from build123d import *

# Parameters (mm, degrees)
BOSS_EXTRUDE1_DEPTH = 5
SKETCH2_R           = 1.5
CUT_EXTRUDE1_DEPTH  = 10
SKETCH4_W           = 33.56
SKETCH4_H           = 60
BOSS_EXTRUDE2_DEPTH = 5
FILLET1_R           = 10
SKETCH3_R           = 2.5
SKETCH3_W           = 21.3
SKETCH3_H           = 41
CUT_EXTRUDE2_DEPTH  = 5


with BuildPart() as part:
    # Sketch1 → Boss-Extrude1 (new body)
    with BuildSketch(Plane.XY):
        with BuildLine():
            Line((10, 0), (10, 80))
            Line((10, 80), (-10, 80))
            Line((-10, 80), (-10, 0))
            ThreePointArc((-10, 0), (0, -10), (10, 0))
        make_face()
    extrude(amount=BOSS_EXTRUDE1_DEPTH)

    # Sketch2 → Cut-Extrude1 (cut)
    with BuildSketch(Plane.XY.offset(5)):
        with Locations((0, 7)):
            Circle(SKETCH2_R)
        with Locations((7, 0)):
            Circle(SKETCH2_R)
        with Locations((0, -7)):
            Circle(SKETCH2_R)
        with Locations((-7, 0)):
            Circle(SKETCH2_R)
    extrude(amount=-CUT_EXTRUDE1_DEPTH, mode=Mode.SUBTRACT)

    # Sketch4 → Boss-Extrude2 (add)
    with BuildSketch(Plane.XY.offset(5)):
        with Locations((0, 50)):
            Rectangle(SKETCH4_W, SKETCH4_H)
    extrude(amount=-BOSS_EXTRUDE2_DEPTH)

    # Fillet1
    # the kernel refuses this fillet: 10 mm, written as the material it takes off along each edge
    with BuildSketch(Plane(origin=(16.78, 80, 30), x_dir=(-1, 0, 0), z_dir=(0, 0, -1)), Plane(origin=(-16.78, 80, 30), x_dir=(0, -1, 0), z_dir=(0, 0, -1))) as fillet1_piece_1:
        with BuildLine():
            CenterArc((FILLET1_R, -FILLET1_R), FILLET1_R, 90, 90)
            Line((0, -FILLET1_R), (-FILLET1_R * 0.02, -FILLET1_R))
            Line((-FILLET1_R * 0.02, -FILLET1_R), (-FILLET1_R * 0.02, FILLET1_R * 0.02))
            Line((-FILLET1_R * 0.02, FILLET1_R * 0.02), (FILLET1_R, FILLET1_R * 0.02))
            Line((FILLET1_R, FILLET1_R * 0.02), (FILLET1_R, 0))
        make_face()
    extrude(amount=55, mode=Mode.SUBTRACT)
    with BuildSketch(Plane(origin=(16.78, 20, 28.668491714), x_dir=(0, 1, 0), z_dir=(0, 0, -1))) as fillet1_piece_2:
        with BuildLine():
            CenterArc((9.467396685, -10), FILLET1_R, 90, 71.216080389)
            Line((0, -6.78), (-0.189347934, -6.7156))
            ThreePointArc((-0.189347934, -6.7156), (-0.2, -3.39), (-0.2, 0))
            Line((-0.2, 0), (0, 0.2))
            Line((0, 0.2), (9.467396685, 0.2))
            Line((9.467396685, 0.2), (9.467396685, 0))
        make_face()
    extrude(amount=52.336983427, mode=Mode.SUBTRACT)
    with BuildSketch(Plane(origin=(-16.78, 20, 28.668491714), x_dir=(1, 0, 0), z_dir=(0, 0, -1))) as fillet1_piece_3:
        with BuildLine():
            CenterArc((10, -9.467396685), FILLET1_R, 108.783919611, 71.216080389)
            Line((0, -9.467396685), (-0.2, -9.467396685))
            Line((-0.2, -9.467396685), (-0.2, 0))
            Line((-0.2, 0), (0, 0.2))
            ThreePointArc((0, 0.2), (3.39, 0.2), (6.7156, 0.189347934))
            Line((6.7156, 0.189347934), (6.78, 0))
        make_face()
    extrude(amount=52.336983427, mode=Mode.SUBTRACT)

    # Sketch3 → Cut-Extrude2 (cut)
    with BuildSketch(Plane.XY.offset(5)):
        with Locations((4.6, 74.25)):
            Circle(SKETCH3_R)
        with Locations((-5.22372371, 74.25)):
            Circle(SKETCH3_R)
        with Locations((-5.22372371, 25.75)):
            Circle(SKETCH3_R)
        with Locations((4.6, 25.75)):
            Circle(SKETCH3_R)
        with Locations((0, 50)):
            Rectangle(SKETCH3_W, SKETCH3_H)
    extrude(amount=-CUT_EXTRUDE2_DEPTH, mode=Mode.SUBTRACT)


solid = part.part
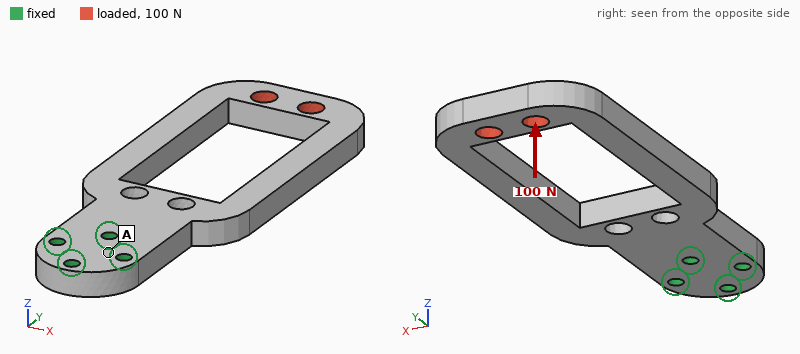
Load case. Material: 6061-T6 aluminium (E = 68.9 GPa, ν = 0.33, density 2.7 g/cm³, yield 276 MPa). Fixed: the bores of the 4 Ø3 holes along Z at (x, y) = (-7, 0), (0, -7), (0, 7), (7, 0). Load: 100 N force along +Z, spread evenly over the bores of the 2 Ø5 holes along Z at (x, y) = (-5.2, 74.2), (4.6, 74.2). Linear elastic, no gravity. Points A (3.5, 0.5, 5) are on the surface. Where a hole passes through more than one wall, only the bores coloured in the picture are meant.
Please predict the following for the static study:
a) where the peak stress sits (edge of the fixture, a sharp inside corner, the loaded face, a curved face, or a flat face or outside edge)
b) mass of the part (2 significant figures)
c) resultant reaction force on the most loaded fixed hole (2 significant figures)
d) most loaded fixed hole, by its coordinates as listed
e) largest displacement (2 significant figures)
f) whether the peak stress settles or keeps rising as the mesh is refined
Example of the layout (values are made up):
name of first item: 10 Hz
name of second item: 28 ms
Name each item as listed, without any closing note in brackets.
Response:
where the peak stress sits: edge of the fixture
mass of the part: 20 g
resultant reaction force on the most loaded fixed hole: 500 N
most loaded fixed hole, by its coordinates as listed: (0, 7)
largest displacement: 1.1 mm
whether the peak stress settles or keeps rising as the mesh is refined: keeps rising
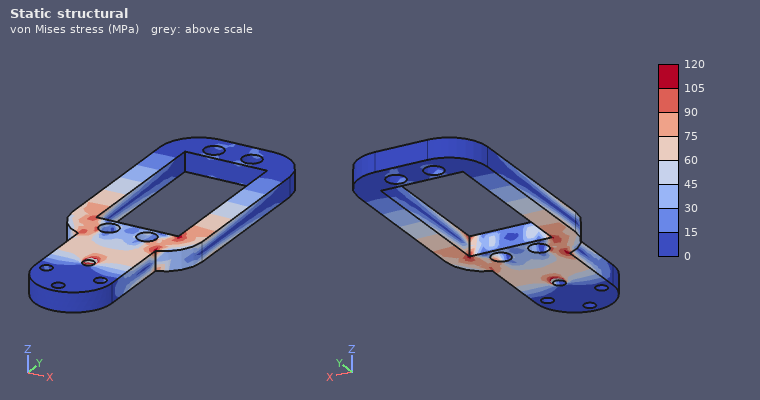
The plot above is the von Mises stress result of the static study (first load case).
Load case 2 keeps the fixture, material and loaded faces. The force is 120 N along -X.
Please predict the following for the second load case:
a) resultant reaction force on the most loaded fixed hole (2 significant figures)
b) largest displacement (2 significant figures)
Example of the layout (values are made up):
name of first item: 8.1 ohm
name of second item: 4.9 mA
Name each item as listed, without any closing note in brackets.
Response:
resultant reaction force on the most loaded fixed hole: 430 N
largest displacement: 0.19 mm
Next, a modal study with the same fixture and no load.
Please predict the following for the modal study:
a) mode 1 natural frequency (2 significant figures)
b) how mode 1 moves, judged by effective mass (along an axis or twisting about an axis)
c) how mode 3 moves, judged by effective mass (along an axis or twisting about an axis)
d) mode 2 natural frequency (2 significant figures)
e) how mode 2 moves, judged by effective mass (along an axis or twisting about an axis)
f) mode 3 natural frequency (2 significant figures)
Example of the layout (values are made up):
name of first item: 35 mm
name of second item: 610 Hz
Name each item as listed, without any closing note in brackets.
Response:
mode 1 natural frequency: 710 Hz
how mode 1 moves, judged by effective mass: along Z
how mode 3 moves, judged by effective mass: twisting about Y
mode 2 natural frequency: 1700 Hz
how mode 2 moves, judged by effective mass: along X
mode 3 natural frequency: 2100 Hz
